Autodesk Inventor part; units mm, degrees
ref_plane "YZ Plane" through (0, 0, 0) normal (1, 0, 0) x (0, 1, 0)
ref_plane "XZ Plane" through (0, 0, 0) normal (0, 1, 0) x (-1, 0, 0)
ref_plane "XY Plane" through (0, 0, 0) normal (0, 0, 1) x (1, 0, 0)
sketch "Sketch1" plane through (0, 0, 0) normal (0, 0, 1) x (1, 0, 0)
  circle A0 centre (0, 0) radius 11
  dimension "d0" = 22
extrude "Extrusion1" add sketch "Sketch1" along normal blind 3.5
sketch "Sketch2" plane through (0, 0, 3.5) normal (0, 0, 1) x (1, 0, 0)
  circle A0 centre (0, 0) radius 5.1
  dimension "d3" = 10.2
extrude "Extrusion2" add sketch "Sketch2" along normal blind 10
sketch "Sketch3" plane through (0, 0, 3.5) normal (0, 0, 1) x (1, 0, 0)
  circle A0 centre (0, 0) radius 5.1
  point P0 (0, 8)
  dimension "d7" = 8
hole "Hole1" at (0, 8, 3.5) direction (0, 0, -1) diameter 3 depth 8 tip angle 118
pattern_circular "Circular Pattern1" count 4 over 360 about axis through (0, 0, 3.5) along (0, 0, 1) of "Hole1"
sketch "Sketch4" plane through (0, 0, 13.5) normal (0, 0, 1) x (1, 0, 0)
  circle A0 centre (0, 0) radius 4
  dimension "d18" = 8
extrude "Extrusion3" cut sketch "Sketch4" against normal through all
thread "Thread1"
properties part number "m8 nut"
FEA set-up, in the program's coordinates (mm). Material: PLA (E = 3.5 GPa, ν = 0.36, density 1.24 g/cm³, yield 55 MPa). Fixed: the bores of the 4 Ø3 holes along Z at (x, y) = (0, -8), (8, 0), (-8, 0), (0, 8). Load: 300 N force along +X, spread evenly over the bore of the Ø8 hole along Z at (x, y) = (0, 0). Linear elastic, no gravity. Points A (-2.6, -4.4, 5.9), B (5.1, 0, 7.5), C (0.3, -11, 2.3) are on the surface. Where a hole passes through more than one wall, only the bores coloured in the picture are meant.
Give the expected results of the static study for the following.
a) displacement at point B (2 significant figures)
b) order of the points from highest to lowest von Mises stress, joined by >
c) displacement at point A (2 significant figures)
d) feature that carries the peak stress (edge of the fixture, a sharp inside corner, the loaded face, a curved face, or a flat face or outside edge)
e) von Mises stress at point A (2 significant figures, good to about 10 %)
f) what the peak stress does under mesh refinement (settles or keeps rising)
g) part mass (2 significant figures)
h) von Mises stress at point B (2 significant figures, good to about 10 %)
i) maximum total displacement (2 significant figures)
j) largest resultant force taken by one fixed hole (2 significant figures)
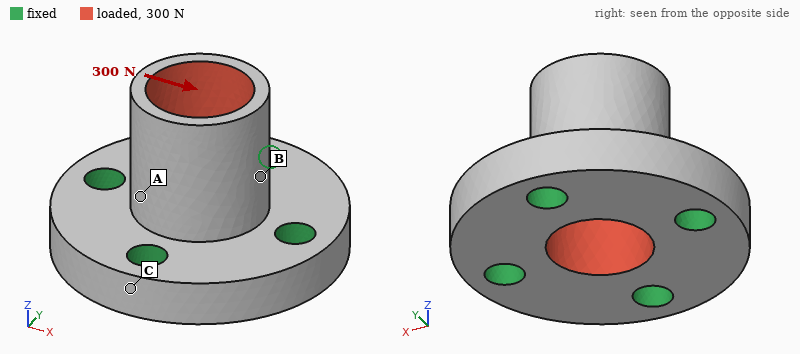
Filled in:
0.068 mm
A > B > C
0.040 mm
a sharp inside corner
12 MPa
keeps rising
1.7 g
5.3 MPa
0.12 mm
140 N
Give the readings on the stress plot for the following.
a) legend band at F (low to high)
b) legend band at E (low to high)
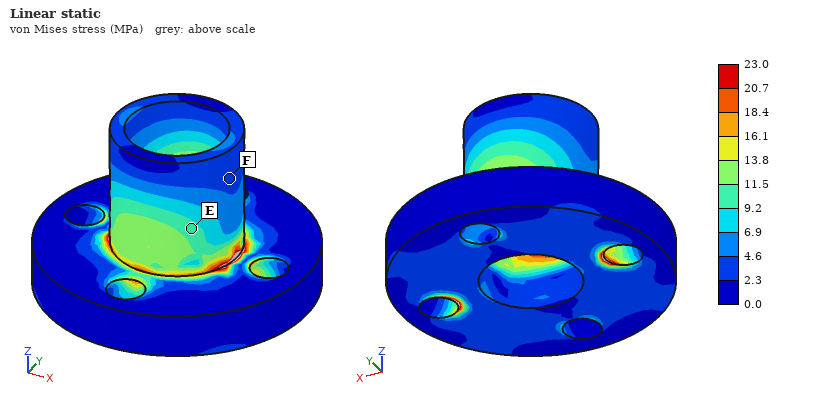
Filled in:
2.3 to 4.6 MPa
9.2 to 11.5 MPa
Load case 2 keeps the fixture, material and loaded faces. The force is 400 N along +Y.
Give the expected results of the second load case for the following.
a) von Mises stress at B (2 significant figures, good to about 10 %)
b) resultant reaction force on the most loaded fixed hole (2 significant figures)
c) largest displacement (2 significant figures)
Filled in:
17 MPa
180 N
0.16 mm
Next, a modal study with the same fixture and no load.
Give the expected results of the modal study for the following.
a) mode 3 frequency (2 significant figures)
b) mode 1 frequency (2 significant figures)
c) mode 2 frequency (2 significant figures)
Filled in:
14 kHz
13 kHz
13 kHz
